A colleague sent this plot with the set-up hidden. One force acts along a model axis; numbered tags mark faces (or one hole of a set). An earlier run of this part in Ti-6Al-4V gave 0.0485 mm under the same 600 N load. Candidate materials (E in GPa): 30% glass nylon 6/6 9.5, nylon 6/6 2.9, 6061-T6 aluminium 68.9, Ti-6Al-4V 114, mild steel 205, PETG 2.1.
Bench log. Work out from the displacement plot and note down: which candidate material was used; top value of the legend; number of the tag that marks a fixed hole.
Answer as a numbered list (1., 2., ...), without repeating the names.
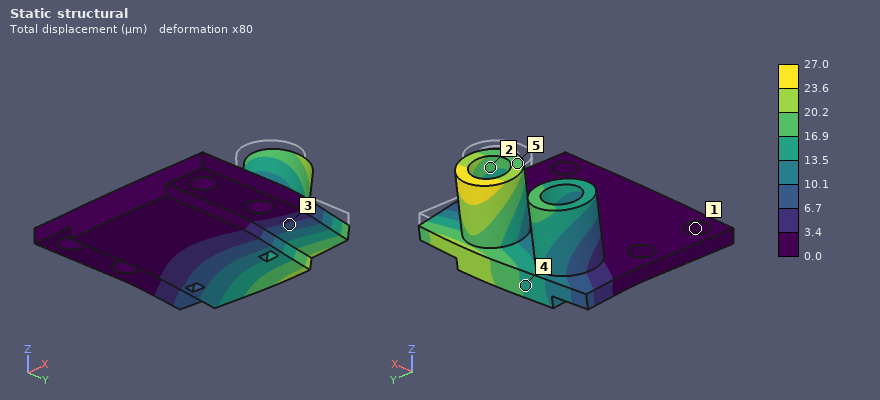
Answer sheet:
1. mild steel
2. 27.0 µm
3. 1
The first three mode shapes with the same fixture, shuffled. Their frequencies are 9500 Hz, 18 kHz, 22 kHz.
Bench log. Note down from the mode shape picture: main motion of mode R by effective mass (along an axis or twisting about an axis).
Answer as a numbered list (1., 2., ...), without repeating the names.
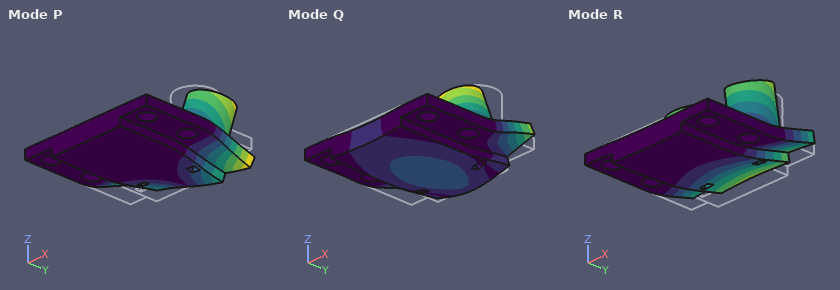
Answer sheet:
1. along Z
